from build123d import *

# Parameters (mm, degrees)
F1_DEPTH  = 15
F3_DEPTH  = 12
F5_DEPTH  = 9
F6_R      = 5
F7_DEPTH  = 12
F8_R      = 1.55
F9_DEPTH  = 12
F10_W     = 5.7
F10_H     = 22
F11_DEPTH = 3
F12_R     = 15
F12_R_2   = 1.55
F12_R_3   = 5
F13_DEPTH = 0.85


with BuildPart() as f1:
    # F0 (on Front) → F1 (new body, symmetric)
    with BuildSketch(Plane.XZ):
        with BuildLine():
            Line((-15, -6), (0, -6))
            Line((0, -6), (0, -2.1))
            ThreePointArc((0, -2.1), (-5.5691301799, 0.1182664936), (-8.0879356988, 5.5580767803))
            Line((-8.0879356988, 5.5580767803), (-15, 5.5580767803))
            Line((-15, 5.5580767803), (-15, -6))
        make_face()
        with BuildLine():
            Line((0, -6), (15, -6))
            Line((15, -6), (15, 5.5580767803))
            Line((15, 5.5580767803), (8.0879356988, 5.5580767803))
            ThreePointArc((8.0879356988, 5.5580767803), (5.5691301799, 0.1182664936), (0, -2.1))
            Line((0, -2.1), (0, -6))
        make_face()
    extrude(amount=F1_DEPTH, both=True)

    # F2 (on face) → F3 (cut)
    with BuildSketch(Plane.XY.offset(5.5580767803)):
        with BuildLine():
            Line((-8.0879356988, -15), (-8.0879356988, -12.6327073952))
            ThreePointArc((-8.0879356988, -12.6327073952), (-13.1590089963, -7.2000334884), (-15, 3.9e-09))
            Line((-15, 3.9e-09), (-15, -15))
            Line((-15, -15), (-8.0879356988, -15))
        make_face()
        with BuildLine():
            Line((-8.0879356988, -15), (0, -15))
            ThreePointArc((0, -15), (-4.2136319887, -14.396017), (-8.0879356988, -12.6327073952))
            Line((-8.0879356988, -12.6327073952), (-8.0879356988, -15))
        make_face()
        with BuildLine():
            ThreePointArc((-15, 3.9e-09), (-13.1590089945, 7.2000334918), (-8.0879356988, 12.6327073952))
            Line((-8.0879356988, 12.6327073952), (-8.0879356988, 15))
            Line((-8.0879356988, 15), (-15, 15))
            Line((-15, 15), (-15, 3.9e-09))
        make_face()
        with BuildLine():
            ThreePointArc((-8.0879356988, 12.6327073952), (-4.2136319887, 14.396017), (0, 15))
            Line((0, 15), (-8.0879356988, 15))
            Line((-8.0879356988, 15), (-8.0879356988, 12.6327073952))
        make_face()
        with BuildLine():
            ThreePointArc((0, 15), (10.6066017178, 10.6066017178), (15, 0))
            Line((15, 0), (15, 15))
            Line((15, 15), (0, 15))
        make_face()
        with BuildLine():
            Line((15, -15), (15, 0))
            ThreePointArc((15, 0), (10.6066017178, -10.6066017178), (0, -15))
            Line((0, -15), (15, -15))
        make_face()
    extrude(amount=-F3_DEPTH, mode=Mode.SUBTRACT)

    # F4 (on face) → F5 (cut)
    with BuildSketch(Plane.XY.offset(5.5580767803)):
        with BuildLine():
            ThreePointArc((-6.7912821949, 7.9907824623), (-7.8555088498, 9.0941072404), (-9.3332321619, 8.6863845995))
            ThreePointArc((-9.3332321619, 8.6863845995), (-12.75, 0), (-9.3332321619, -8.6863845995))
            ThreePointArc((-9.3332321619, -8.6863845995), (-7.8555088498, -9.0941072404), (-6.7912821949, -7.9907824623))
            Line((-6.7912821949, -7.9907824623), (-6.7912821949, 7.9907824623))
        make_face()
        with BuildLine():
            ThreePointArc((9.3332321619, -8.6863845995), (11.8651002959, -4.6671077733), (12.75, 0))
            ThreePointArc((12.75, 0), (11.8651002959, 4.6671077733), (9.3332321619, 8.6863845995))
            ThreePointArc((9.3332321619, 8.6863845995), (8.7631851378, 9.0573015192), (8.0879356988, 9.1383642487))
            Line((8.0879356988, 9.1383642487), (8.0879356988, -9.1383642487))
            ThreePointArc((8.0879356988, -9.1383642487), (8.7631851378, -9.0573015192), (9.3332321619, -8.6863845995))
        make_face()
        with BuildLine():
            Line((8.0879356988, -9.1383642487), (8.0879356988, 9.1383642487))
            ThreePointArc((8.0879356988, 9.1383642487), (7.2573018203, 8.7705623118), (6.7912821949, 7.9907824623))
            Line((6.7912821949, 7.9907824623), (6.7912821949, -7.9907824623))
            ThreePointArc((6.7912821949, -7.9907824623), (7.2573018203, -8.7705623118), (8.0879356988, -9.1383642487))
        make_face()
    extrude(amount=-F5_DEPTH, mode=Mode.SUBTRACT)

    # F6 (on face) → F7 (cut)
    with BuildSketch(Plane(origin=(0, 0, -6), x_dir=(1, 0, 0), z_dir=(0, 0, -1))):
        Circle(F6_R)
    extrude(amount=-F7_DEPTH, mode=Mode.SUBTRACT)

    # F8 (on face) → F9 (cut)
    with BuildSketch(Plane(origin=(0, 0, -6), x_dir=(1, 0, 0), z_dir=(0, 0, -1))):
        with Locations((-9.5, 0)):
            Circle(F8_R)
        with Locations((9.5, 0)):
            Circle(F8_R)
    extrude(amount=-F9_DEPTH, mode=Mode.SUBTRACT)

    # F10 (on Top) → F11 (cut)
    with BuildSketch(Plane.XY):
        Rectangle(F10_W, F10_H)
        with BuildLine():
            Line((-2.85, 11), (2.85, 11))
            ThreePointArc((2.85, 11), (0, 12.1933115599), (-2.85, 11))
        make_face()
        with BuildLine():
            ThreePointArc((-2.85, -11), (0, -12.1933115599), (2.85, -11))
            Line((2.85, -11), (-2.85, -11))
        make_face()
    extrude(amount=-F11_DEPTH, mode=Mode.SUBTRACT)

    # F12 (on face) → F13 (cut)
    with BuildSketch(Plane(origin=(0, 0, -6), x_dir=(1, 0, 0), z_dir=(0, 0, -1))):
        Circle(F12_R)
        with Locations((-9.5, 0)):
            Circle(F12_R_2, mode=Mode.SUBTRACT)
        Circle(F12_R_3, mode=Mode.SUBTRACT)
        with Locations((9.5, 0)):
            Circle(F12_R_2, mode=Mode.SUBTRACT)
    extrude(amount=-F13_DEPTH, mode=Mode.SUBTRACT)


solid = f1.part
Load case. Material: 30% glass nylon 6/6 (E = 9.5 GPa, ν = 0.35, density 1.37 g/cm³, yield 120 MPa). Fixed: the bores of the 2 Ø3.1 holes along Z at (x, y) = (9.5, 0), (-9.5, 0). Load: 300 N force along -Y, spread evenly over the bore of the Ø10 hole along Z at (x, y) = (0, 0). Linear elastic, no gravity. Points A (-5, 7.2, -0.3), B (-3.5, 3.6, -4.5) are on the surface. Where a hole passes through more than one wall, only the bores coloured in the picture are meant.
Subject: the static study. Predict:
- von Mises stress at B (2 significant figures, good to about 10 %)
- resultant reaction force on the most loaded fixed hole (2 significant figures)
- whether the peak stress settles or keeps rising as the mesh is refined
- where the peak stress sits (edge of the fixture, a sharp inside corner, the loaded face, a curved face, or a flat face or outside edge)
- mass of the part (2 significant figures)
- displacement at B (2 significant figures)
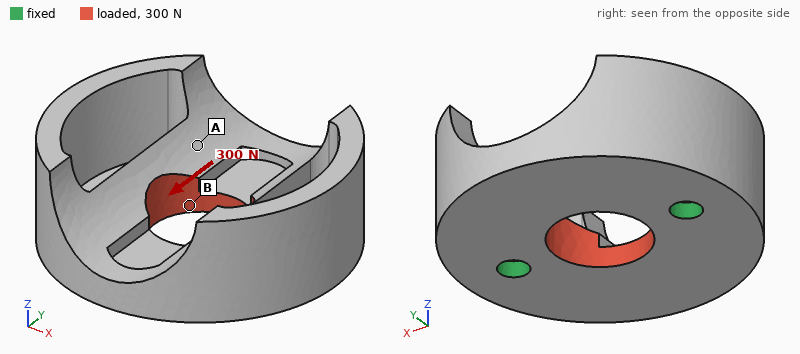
4.7 MPa
150 N
keeps rising
edge of the fixture
4.1 g
9.9 µm
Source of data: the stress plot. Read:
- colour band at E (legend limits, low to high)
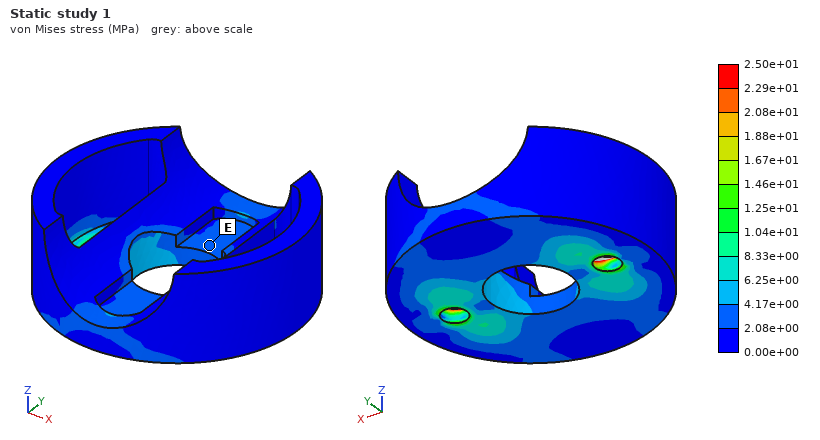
2.08e+00 to 4.17e+00 MPa
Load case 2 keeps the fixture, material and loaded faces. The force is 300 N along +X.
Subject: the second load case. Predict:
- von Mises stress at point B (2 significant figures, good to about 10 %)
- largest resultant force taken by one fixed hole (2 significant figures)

7.1 MPa
150 N
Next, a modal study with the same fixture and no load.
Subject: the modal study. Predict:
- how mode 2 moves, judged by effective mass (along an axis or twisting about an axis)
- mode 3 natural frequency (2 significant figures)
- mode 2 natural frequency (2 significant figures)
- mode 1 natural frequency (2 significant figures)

along Z
7600 Hz
6500 Hz
3300 Hz
